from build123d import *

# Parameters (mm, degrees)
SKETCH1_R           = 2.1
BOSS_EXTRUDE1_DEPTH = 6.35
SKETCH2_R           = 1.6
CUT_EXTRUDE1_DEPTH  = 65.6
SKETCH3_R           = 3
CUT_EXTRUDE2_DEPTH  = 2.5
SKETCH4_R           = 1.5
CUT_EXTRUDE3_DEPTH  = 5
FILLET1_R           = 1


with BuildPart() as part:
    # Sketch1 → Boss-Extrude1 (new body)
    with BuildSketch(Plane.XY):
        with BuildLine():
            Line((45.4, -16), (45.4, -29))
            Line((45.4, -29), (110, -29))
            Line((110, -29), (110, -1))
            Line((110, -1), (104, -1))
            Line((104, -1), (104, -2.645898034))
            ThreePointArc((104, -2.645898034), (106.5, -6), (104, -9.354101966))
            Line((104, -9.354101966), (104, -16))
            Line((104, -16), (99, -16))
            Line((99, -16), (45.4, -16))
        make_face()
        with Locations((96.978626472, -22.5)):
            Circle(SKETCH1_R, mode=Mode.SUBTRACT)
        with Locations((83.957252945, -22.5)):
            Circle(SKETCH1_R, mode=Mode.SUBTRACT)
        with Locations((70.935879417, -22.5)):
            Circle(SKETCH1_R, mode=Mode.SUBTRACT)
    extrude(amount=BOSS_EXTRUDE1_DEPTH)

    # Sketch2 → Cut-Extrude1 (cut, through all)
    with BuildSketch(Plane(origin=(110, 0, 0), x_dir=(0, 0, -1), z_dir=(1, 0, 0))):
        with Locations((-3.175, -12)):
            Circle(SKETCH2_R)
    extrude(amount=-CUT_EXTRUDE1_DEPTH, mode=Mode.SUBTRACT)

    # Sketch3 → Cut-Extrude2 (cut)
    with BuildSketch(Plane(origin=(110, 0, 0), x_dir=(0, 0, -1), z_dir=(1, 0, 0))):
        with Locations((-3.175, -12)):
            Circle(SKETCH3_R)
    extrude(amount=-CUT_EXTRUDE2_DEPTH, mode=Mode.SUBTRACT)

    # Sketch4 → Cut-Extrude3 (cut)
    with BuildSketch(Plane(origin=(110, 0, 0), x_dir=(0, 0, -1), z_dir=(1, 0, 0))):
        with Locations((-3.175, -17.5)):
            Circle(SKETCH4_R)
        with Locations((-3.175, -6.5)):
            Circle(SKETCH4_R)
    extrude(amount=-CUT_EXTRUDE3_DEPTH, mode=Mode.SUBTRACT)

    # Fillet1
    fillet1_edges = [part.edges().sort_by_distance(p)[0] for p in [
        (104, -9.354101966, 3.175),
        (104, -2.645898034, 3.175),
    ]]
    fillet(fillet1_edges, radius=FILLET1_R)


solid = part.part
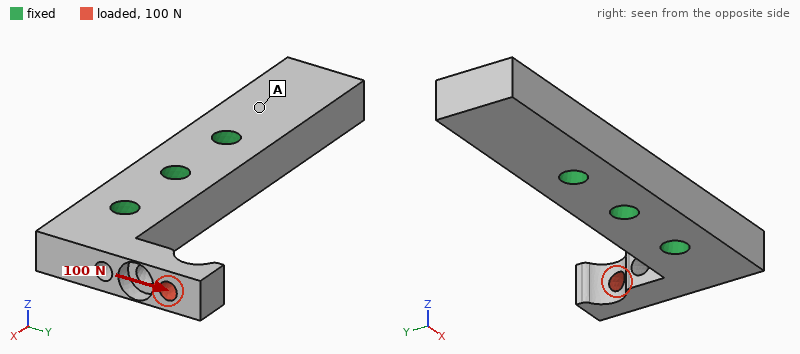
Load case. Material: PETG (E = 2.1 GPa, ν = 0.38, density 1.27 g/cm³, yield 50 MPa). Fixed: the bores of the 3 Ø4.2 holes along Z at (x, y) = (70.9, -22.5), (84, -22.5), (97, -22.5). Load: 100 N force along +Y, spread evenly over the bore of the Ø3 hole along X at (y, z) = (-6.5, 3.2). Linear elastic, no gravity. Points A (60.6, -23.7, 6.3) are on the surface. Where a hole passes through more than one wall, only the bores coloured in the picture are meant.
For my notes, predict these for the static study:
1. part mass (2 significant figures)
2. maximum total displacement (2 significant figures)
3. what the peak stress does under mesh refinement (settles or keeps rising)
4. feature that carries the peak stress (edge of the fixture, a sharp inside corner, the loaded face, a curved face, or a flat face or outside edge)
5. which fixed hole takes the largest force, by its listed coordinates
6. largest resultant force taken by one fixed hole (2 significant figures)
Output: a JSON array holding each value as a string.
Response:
["6.9 g", "0.49 mm", "keeps rising", "a sharp inside corner", "(97, -22.5)", "140 N"]
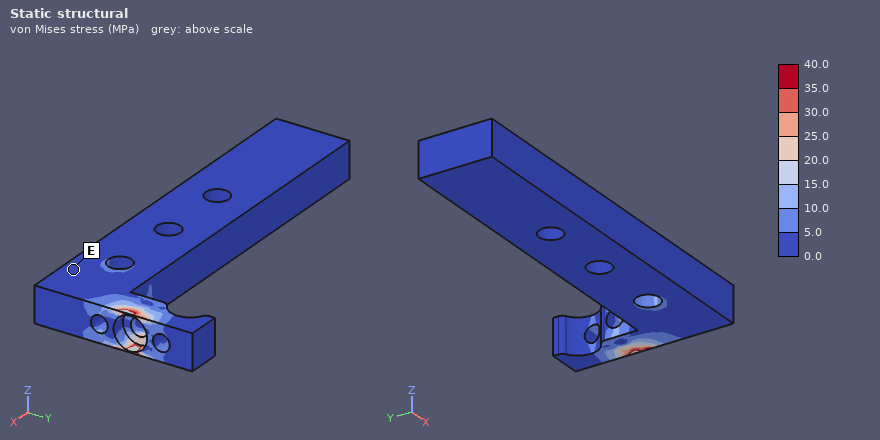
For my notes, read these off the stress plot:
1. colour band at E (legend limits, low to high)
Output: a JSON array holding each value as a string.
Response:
["0.0 to 5.0 MPa"]
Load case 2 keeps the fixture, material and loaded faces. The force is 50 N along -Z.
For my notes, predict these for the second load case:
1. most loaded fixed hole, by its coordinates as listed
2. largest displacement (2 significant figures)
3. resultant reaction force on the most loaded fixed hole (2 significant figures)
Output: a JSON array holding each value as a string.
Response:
["(97, -22.5)", "0.73 mm", "57 N"]
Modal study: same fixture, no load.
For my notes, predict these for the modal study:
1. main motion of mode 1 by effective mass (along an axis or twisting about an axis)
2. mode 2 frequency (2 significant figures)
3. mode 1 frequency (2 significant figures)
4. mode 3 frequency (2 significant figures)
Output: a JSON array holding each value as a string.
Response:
["along Z", "2400 Hz", "2000 Hz", "2500 Hz"]
